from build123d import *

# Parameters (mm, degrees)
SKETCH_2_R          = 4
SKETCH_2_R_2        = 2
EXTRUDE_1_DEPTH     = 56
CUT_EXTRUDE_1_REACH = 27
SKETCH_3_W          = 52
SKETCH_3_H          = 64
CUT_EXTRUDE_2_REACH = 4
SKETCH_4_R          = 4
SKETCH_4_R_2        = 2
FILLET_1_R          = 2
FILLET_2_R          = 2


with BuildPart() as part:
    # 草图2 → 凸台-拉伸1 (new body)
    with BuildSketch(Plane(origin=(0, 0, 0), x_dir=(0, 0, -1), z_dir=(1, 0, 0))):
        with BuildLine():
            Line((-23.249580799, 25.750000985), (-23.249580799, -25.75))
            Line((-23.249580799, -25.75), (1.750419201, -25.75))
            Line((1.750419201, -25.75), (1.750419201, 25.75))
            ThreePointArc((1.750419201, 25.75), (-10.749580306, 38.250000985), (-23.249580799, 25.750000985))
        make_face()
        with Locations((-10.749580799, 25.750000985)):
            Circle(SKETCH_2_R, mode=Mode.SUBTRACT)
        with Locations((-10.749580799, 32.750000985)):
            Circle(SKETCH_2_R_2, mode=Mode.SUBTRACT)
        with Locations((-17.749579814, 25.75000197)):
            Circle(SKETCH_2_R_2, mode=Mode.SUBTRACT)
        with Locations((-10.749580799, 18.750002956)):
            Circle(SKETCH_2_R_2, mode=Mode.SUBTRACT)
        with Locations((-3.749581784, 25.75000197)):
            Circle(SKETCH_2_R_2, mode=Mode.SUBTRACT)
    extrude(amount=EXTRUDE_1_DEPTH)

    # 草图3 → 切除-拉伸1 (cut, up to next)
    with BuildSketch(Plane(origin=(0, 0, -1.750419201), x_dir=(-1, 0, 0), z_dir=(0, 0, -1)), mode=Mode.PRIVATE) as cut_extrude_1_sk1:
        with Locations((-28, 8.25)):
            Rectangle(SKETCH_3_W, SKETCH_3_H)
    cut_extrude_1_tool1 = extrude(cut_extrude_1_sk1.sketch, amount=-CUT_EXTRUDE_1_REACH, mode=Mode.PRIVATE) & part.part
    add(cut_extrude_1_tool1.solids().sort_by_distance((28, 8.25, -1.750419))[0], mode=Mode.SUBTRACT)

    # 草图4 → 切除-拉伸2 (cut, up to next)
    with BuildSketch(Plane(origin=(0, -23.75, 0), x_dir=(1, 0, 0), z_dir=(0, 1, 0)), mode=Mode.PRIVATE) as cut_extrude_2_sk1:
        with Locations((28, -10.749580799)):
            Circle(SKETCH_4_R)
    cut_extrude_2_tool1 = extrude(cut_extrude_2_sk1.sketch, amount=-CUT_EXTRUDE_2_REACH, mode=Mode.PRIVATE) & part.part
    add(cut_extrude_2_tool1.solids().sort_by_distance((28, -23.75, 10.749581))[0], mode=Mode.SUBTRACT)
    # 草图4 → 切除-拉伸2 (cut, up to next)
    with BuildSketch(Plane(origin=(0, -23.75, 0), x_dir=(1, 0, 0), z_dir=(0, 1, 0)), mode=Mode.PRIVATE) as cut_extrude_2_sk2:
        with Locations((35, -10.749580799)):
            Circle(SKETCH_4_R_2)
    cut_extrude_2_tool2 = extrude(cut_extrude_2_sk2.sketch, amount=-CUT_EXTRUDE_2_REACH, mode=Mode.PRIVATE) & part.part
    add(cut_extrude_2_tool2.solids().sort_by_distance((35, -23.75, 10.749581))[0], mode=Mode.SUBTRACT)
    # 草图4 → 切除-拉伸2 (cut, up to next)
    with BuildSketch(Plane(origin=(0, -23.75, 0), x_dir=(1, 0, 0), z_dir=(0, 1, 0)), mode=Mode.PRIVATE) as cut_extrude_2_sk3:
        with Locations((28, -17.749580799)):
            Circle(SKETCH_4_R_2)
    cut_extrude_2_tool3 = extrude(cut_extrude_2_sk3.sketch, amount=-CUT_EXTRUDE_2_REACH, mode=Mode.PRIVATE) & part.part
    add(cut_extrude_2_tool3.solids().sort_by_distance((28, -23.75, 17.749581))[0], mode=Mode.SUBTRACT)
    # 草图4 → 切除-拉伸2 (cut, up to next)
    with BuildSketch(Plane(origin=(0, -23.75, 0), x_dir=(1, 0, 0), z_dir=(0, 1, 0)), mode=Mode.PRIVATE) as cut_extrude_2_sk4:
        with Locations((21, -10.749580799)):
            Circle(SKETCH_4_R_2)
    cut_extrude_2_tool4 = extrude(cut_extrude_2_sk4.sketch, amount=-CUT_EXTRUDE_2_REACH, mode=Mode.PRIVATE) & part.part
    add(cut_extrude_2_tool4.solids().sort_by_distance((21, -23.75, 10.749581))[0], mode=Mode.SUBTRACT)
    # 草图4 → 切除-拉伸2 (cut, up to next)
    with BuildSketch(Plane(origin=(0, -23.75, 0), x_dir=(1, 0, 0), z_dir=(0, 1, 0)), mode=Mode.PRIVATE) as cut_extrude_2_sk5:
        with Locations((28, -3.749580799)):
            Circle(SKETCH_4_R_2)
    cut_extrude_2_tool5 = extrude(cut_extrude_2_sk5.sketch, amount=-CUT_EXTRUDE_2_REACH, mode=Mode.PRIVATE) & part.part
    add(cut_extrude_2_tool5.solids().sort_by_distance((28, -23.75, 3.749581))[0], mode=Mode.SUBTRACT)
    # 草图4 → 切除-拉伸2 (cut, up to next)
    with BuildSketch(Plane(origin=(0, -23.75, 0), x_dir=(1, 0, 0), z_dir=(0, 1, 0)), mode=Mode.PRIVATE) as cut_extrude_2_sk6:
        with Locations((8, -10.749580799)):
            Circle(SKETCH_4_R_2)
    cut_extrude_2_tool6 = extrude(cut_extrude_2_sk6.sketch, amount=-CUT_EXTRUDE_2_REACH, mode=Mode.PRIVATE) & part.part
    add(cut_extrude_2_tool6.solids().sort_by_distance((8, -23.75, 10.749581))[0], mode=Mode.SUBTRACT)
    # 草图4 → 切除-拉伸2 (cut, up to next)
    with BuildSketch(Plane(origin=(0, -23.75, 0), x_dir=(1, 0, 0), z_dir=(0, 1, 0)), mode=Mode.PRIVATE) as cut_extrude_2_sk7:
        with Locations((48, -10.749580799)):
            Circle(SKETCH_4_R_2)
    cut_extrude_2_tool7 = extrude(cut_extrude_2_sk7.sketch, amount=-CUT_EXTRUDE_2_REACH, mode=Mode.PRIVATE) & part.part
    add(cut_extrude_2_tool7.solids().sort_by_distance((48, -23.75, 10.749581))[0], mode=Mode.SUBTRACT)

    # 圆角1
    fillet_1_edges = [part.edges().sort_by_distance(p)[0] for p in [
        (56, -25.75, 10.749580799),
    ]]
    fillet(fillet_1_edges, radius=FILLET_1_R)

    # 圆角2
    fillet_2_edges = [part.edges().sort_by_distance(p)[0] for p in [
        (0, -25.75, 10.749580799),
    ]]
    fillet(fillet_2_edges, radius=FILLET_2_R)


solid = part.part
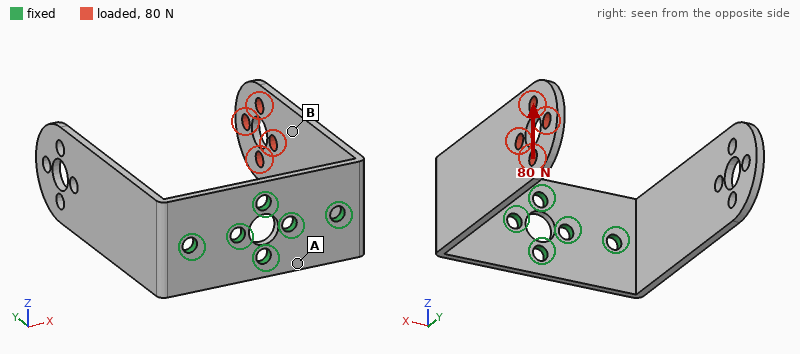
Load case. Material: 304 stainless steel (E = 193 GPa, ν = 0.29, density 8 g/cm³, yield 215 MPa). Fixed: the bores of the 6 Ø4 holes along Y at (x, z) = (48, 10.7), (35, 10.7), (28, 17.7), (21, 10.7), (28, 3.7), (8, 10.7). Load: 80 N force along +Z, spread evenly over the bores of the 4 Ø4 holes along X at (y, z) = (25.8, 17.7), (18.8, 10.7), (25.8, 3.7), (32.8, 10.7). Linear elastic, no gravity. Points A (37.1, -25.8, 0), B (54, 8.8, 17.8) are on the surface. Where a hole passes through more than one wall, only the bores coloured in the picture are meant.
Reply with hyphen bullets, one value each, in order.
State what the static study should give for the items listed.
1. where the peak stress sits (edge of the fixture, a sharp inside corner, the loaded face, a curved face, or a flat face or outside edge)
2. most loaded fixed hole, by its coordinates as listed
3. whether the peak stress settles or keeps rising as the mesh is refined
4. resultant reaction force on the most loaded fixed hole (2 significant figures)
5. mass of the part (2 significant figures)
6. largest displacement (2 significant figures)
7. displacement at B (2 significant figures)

- edge of the fixture
- (48, 10.7)
- keeps rising
- 88 N
- 64 g
- 0.28 mm
- 0.15 mm
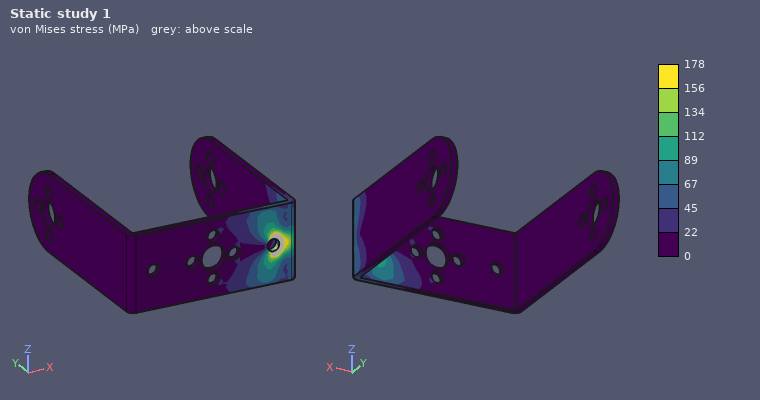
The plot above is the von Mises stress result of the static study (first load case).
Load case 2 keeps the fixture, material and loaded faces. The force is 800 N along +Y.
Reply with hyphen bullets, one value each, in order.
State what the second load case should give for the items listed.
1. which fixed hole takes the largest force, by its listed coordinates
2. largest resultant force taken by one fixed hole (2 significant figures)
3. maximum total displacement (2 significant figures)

- (48, 10.7)
- 890 N
- 0.36 mm
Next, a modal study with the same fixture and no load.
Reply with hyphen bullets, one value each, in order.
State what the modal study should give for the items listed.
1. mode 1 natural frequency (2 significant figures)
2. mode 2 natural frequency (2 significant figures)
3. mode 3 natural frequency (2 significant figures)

- 400 Hz
- 400 Hz
- 940 Hz
